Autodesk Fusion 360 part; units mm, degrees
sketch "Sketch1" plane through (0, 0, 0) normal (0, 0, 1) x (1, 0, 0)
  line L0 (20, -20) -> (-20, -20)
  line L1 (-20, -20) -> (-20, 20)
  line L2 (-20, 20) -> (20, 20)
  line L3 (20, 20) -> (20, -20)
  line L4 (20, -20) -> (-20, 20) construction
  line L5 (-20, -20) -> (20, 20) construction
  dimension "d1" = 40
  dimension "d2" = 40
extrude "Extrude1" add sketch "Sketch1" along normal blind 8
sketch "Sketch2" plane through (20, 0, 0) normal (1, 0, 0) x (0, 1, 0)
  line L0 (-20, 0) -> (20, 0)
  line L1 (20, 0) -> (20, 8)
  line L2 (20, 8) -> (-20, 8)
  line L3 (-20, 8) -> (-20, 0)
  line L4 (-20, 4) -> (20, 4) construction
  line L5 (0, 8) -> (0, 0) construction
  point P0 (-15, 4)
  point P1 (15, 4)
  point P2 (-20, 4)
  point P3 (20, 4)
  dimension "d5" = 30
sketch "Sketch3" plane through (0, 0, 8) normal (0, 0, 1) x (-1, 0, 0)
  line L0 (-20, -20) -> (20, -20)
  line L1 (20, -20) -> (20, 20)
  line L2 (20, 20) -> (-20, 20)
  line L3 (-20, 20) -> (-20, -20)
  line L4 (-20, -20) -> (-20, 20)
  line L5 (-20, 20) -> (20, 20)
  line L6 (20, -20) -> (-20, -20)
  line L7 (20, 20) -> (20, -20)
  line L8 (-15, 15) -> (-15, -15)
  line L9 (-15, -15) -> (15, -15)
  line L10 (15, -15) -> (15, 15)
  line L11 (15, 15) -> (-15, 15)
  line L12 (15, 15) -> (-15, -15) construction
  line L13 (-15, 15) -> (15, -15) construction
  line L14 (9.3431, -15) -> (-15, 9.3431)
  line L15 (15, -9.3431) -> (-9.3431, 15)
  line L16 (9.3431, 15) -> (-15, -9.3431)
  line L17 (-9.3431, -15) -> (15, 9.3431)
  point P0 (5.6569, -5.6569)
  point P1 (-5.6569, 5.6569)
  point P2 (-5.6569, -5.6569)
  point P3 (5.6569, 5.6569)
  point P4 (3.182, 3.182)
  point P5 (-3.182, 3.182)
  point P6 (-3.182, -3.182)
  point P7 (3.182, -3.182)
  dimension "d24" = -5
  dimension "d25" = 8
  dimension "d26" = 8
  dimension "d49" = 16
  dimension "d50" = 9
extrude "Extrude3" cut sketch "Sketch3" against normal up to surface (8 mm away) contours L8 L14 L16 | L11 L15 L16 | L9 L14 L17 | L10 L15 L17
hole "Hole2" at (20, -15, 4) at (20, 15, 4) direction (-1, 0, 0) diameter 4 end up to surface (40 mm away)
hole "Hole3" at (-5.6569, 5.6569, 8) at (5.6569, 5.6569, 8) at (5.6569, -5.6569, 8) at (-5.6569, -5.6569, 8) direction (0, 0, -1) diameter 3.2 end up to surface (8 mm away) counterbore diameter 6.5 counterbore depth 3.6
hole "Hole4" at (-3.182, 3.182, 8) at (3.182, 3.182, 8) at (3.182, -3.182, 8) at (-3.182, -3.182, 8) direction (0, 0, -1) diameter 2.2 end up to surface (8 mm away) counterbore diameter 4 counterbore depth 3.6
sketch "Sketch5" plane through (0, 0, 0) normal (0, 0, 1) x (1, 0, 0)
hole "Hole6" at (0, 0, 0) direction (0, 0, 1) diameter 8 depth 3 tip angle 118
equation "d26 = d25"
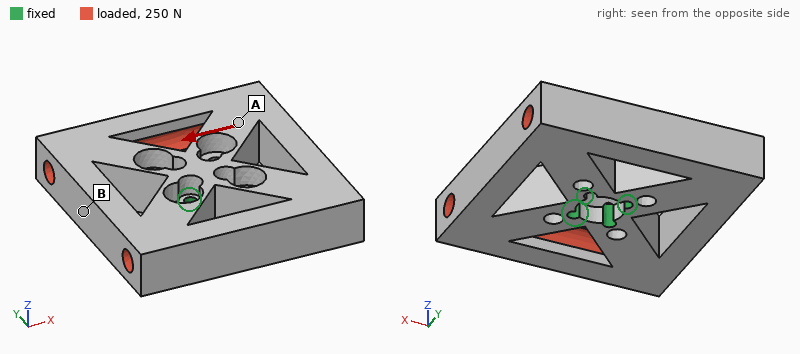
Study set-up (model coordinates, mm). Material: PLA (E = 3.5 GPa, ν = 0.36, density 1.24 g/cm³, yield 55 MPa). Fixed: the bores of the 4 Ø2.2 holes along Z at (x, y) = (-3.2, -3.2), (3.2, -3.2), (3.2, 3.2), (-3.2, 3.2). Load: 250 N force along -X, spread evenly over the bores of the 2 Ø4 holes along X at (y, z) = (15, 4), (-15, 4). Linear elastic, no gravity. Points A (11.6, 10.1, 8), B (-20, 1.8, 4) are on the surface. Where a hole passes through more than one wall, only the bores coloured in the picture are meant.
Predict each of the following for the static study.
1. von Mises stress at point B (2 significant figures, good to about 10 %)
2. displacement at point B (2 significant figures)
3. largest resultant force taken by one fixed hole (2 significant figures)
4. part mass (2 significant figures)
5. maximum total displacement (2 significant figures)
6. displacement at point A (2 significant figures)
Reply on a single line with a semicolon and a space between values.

1.2 MPa; 32 µm; 65 N; 10 g; 44 µm; 27 µm
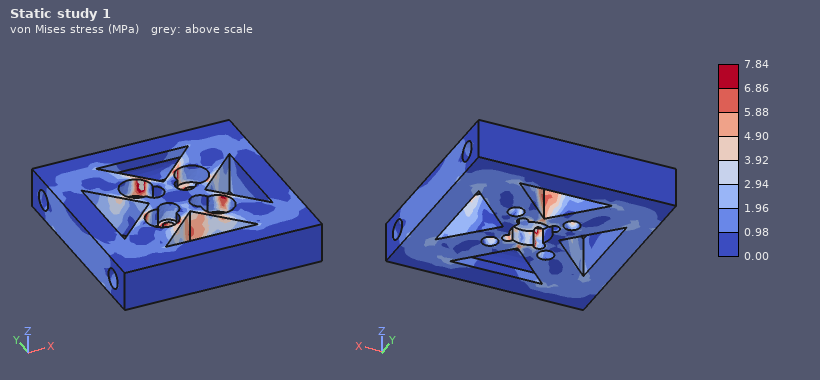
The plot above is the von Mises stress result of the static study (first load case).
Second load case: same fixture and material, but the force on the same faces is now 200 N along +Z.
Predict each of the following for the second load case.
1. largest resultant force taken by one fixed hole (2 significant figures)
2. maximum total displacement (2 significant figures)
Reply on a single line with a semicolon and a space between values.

64 N; 0.13 mm
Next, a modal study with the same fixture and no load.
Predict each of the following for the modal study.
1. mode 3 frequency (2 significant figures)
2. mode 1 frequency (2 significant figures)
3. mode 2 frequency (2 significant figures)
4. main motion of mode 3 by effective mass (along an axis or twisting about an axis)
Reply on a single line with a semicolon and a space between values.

2400 Hz; 2000 Hz; 2100 Hz; twisting about Z
